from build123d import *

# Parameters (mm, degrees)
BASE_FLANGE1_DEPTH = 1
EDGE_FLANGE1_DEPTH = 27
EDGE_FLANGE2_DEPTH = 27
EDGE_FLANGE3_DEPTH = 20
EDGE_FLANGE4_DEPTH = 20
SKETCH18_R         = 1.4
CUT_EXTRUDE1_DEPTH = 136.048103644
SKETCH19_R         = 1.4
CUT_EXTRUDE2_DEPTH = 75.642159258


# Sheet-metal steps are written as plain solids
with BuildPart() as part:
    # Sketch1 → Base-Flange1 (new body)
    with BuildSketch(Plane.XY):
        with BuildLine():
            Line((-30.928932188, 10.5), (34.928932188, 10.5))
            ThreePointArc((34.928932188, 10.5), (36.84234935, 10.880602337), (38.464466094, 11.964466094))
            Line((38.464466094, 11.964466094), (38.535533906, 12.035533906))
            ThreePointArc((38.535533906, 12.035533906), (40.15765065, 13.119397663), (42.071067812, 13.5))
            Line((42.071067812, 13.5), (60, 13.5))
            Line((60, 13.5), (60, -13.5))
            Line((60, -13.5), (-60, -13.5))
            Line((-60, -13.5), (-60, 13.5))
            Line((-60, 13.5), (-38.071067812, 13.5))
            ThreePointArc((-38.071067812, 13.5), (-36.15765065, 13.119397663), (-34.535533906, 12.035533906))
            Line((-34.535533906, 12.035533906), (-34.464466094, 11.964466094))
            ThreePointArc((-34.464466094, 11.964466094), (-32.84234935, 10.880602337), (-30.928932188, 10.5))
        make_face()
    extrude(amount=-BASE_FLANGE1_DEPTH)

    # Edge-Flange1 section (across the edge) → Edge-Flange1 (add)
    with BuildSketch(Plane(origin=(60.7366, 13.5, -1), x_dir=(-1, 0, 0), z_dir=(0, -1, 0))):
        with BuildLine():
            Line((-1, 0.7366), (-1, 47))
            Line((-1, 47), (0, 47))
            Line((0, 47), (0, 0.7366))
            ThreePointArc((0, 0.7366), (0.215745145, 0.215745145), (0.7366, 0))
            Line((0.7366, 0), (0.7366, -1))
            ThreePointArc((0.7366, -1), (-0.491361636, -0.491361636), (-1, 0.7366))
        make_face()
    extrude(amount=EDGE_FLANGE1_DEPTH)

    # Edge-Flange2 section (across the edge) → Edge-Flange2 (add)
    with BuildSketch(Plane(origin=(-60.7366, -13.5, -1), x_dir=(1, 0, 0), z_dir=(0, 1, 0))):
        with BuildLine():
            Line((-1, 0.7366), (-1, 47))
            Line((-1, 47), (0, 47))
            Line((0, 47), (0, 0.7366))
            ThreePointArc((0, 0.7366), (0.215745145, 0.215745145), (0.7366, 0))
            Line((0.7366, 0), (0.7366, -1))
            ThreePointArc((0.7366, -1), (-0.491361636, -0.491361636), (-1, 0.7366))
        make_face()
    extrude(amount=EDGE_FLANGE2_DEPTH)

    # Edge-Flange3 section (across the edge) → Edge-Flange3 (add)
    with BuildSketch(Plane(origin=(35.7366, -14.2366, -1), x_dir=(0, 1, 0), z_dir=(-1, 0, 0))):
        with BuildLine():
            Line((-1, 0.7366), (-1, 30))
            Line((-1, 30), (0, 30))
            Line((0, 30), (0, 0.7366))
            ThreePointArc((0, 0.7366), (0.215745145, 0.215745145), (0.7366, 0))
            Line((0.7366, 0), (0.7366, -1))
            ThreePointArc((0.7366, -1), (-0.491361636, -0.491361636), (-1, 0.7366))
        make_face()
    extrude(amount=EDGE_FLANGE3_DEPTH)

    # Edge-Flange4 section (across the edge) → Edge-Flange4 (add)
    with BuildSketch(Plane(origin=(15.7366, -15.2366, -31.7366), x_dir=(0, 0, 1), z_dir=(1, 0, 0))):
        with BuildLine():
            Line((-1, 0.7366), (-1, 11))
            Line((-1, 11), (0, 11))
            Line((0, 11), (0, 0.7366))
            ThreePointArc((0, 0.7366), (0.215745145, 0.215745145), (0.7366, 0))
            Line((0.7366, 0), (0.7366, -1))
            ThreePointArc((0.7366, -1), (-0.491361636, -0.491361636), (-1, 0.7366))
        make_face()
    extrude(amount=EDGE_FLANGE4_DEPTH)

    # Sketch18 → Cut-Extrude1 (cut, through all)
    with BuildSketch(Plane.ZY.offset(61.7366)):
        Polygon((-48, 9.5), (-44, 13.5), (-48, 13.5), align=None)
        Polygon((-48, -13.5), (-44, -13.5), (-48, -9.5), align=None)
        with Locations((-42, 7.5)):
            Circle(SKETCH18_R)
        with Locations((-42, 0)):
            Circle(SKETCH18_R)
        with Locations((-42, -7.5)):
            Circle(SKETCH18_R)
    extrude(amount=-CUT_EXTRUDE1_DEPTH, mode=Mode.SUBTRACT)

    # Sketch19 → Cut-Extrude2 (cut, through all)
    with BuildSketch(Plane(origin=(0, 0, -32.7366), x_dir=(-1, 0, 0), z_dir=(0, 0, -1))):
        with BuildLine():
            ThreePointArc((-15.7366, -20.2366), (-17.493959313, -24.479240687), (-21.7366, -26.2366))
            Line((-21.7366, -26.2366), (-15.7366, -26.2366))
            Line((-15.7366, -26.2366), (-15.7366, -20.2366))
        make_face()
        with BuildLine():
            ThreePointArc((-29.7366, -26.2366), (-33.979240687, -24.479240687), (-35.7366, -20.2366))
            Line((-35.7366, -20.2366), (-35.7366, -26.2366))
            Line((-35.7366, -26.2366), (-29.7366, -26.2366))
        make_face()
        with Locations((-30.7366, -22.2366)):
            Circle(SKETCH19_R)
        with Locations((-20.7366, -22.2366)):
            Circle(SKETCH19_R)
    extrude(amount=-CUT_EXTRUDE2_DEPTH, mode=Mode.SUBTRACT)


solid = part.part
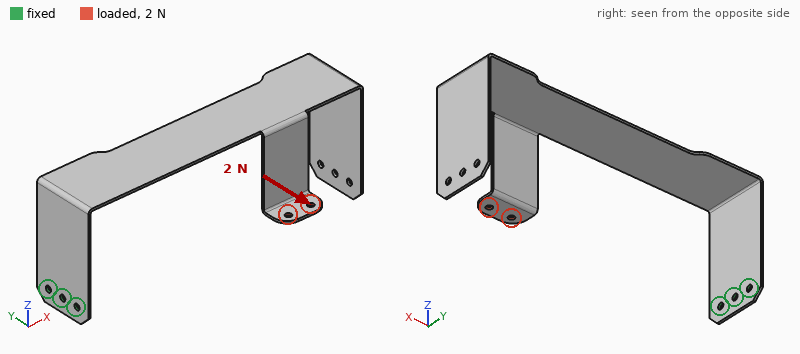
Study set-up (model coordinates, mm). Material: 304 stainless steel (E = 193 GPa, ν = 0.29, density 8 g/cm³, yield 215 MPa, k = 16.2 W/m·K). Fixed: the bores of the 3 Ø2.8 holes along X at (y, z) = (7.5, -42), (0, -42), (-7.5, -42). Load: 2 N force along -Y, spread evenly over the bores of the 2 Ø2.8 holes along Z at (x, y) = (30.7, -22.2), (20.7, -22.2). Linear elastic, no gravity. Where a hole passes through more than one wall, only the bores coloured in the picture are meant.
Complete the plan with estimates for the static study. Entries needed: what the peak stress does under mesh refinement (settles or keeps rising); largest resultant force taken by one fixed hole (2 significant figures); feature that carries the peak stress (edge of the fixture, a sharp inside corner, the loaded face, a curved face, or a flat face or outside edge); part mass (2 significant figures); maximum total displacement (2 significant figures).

keeps rising
9.3 N
edge of the fixture
51 g
1.5 mm
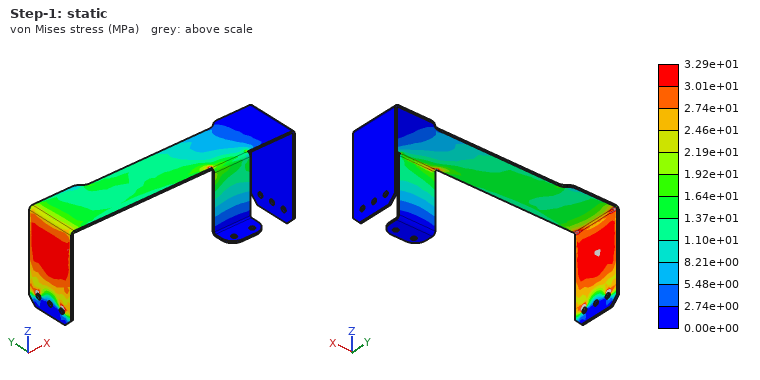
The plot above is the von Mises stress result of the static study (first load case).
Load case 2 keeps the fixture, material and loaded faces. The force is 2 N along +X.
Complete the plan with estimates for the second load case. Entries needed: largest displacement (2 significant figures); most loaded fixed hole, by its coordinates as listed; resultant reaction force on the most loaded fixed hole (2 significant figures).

1.5 mm
(-7.5, -42)
3.2 N
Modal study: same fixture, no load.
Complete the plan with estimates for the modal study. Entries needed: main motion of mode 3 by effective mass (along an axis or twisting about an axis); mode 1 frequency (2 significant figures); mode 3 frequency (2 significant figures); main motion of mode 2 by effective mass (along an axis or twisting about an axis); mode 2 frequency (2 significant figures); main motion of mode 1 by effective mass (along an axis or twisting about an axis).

along X
21 Hz
100 Hz
along Y
39 Hz
along Z
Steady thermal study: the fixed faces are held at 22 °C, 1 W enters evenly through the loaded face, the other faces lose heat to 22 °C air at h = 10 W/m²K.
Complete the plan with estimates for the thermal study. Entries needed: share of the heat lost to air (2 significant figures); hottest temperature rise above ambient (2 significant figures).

100 %
80 K
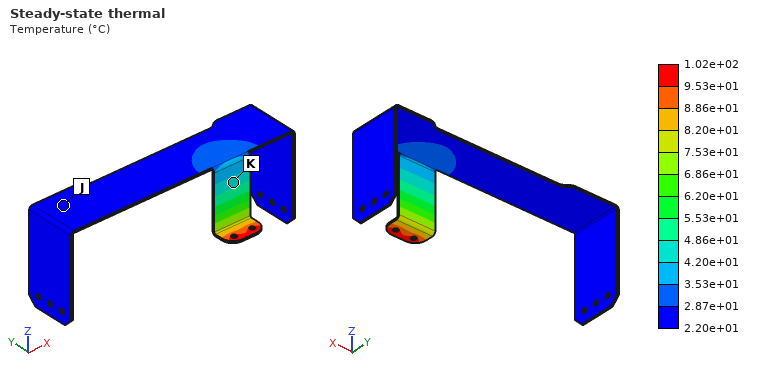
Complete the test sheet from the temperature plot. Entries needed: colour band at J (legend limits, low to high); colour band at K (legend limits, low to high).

2.20e+01 to 2.87e+01 °C
4.20e+01 to 4.86e+01 °C
